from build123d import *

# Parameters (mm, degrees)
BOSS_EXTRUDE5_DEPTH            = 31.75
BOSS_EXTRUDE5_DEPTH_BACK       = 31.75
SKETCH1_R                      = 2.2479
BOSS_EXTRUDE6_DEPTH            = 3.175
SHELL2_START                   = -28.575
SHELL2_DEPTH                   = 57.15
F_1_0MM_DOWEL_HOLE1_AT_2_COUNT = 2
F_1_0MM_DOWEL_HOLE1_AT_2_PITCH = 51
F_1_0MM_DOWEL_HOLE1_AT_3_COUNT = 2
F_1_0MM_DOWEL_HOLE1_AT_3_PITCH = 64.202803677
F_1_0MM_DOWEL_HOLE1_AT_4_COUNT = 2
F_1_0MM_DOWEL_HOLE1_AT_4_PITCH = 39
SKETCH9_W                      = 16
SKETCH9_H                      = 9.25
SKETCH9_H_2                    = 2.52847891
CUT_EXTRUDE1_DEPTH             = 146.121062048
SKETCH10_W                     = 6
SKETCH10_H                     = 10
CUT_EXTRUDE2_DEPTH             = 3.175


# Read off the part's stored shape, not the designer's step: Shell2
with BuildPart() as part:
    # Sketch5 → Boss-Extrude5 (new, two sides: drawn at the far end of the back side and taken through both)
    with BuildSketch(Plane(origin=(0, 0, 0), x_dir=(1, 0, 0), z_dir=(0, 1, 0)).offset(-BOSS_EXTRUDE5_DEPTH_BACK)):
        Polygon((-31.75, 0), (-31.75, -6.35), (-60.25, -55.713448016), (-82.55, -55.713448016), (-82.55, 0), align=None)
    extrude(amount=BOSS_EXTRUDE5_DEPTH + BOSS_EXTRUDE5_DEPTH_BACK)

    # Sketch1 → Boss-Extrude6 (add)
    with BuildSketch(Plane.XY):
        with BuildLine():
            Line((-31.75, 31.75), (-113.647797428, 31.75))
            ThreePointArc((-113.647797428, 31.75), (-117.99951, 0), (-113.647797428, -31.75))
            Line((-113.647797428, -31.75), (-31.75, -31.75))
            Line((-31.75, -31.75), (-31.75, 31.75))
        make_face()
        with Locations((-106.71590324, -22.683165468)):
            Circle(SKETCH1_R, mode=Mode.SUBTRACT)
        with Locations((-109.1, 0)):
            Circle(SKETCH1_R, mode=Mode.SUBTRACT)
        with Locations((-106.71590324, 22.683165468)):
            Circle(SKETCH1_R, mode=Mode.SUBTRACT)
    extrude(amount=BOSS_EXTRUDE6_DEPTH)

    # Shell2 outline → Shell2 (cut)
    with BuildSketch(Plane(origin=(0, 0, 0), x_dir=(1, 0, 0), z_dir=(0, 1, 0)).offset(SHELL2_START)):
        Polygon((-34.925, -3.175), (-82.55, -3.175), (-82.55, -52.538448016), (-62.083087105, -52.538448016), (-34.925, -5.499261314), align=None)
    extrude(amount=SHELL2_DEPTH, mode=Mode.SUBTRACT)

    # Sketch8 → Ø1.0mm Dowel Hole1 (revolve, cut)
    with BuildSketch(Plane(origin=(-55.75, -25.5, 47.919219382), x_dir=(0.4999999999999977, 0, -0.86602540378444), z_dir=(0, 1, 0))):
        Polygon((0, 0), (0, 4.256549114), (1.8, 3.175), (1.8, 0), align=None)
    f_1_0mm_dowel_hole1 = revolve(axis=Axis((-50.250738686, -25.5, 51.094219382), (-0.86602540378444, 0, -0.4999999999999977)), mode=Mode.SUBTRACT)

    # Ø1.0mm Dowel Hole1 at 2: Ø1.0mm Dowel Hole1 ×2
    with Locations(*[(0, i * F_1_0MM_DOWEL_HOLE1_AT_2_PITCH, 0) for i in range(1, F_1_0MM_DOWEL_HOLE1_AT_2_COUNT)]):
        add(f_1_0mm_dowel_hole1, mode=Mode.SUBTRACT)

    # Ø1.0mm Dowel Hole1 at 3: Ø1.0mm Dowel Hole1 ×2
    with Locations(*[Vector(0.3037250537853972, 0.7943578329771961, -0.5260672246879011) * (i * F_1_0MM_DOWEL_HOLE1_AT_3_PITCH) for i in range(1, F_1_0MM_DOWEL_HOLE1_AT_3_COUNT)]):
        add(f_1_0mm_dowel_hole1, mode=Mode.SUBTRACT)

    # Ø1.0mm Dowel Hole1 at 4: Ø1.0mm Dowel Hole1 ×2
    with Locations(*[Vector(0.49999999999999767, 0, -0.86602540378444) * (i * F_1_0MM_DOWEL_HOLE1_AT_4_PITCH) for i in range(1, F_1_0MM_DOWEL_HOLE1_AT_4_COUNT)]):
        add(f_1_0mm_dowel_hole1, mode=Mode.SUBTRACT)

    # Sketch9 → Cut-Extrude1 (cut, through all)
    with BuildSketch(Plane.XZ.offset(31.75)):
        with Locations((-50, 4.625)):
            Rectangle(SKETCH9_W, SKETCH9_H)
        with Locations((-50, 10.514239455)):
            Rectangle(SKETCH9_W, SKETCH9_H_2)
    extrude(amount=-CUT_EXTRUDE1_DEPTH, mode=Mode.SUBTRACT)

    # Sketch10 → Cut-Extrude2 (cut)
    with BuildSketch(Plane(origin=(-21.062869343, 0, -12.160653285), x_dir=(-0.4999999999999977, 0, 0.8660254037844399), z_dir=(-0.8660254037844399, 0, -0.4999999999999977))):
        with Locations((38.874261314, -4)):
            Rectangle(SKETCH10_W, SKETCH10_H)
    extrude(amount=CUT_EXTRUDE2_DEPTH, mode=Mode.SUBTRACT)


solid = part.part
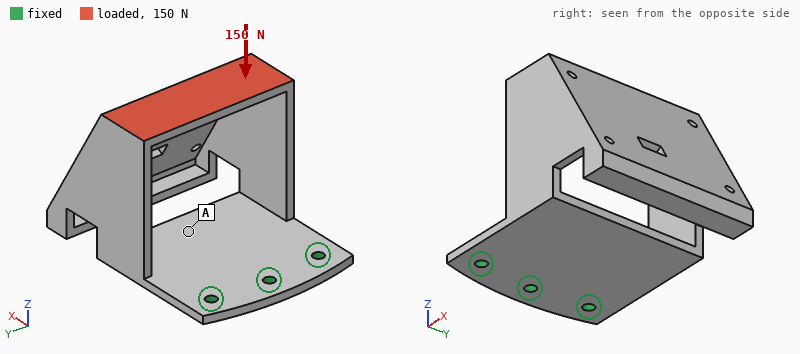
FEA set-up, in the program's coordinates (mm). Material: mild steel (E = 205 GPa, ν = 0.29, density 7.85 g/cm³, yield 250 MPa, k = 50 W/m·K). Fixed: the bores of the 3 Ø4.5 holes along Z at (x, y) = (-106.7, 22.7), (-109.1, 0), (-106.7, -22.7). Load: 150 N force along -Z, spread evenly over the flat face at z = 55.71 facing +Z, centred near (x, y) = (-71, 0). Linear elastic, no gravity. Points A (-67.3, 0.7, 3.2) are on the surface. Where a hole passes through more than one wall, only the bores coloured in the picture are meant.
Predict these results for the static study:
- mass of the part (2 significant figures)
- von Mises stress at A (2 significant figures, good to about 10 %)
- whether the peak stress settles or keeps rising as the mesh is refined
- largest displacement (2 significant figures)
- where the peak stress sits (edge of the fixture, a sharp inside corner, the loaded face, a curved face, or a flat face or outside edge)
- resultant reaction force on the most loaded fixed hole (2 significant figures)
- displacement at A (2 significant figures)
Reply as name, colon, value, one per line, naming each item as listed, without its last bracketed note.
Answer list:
mass of the part: 310 g
von Mises stress at A: 6.3 MPa
whether the peak stress settles or keeps rising as the mesh is refined: keeps rising
largest displacement: 0.17 mm
where the peak stress sits: edge of the fixture
resultant reaction force on the most loaded fixed hole: 71 N
displacement at A: 0.070 mm
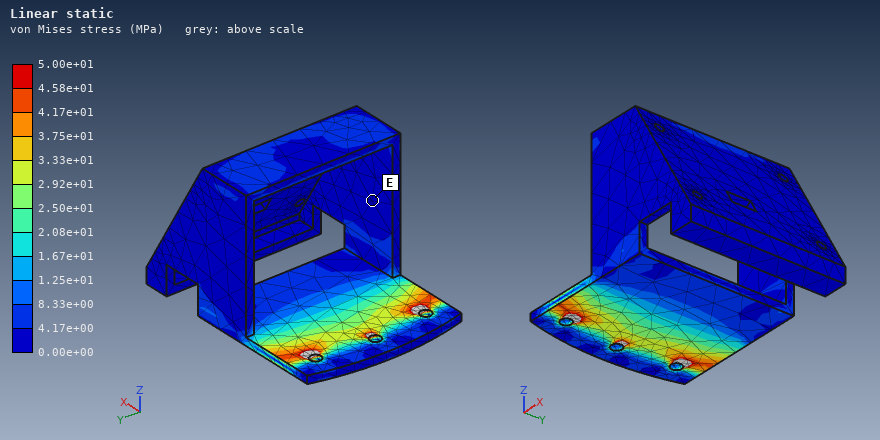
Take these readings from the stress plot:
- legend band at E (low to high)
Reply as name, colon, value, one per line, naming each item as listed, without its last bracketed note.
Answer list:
legend band at E: 0.00e+00 to 4.17e+00 MPa
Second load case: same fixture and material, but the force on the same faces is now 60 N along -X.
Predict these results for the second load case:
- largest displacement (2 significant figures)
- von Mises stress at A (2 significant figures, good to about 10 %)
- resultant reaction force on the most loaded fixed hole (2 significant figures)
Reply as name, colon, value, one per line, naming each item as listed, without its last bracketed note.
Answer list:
largest displacement: 0.19 mm
von Mises stress at A: 5.9 MPa
resultant reaction force on the most loaded fixed hole: 28 N
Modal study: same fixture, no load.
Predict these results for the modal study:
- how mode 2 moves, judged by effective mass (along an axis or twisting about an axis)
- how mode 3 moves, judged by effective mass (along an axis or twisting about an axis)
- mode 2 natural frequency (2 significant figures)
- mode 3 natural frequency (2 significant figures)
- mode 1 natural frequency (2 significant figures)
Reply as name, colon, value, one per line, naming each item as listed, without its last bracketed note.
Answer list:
how mode 2 moves, judged by effective mass: along Y
how mode 3 moves, judged by effective mass: along Y
mode 2 natural frequency: 490 Hz
mode 3 natural frequency: 1100 Hz
mode 1 natural frequency: 220 Hz
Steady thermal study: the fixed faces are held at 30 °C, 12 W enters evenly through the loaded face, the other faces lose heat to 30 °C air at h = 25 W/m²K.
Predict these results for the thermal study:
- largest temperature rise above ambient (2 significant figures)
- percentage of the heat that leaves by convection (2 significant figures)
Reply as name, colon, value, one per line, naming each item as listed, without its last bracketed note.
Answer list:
largest temperature rise above ambient: 41 K
percentage of the heat that leaves by convection: 83 %
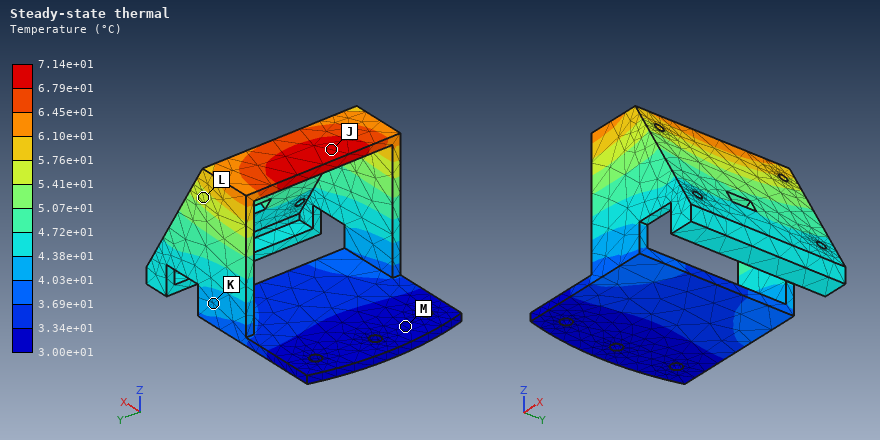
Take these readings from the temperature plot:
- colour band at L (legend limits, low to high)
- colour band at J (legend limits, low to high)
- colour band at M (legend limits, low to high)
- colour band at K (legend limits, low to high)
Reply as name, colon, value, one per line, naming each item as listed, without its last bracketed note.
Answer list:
colour band at L: 5.41e+01 to 5.76e+01 °C
colour band at J: 6.79e+01 to 7.14e+01 °C
colour band at M: 3.00e+01 to 3.34e+01 °C
colour band at K: 4.03e+01 to 4.38e+01 °C
